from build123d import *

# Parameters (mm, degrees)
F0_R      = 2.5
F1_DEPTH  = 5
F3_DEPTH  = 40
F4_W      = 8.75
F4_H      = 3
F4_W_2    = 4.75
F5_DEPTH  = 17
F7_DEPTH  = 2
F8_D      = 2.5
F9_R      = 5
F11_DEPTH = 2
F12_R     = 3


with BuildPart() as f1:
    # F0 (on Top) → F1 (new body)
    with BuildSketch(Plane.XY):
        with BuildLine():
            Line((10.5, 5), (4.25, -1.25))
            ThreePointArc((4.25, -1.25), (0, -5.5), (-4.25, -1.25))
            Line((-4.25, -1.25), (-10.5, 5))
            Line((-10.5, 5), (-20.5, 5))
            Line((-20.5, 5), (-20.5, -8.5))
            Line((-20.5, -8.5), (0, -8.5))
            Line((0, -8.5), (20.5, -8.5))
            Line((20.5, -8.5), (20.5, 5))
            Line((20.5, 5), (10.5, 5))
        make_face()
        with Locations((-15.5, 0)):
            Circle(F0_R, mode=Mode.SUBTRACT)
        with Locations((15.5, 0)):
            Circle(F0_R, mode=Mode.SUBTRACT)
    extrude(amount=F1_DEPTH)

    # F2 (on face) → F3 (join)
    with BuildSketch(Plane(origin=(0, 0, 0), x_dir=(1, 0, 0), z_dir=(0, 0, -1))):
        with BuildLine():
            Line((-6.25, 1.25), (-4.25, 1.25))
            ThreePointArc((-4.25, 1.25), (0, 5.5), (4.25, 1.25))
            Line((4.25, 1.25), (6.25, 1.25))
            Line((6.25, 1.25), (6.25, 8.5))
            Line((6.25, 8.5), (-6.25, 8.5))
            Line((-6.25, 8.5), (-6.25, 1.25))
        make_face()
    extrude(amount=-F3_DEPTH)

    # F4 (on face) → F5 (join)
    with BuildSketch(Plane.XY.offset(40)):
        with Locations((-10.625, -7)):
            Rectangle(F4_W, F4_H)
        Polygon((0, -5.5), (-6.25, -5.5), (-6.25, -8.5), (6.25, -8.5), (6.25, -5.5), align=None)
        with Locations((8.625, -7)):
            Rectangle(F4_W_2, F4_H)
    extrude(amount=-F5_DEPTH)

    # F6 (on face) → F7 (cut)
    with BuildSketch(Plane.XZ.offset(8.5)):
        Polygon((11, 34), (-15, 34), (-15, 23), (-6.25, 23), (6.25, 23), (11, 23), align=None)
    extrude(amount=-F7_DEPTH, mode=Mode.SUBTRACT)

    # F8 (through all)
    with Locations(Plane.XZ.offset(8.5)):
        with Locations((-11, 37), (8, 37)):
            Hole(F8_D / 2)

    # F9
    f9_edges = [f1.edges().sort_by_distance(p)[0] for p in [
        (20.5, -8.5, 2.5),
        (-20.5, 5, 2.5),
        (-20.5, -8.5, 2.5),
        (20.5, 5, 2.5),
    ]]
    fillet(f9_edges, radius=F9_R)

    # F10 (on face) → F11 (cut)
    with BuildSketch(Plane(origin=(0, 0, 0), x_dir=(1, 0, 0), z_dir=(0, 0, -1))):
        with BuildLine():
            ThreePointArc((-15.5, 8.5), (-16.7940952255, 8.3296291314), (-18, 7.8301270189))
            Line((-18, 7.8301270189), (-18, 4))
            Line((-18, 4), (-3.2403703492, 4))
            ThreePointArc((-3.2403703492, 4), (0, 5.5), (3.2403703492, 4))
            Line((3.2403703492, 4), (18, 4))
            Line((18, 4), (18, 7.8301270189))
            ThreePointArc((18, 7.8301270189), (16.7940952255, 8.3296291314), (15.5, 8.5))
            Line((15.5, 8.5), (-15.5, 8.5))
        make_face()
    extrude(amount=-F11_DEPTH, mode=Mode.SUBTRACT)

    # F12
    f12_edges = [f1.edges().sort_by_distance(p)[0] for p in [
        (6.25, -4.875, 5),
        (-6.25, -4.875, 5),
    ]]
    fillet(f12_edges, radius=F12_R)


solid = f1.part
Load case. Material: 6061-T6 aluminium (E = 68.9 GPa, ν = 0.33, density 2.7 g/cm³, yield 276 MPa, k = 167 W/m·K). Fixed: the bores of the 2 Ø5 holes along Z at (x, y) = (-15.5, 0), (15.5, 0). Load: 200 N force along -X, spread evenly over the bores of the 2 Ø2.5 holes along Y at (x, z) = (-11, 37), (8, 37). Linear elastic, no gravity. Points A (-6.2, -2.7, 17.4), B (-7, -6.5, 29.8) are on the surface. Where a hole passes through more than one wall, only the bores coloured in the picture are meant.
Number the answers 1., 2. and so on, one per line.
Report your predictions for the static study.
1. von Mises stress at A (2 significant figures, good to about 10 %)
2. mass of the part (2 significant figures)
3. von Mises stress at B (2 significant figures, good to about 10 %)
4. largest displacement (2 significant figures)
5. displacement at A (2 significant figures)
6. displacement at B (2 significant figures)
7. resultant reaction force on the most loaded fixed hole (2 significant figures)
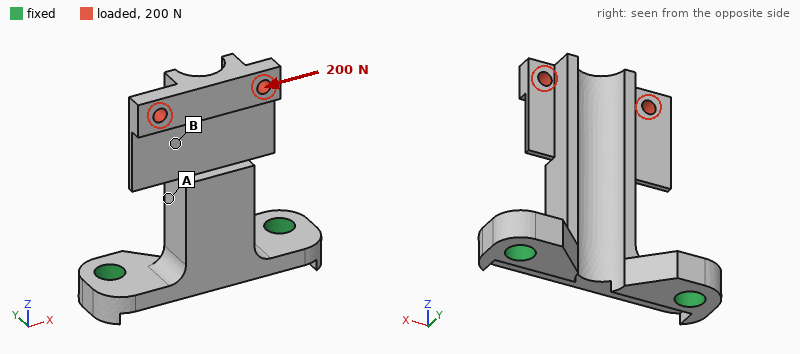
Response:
1. 26 MPa
2. 10 g
3. 9.3 MPa
4. 99 µm
5. 27 µm
6. 60 µm
7. 380 N
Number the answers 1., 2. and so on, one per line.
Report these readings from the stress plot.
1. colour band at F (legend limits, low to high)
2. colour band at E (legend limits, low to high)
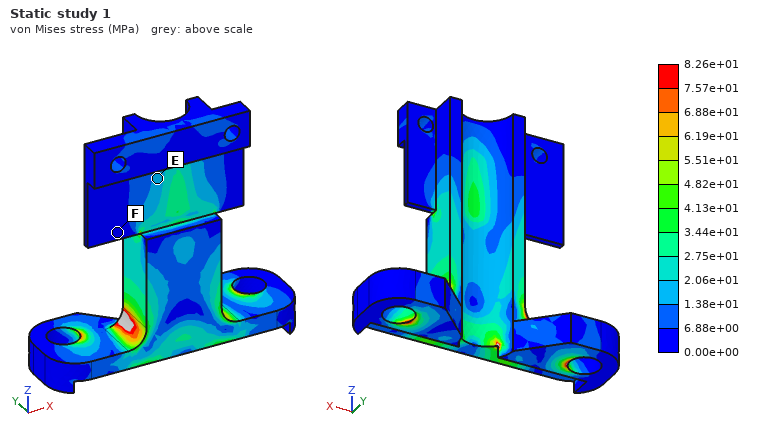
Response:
1. 0.00e+00 to 6.88e+00 MPa
2. 1.38e+01 to 2.06e+01 MPa
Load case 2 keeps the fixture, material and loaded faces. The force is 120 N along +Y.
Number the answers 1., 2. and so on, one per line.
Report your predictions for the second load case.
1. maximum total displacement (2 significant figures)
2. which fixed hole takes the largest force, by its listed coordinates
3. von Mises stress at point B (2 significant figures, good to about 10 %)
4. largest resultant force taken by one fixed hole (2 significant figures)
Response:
1. 0.30 mm
2. (-15.5, 0)
3. 16 MPa
4. 69 N
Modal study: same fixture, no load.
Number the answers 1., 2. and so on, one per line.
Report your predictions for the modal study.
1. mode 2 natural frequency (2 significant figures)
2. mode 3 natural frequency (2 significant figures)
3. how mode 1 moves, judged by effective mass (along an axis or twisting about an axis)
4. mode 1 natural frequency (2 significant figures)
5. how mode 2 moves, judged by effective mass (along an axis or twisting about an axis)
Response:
1. 4600 Hz
2. 5500 Hz
3. along Y
4. 2200 Hz
5. along X
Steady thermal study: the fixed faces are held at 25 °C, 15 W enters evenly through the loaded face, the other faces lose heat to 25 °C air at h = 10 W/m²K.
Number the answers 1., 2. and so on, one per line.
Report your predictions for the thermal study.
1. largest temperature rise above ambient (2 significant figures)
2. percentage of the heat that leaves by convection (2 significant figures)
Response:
1. 71 K
2. 6.4 %
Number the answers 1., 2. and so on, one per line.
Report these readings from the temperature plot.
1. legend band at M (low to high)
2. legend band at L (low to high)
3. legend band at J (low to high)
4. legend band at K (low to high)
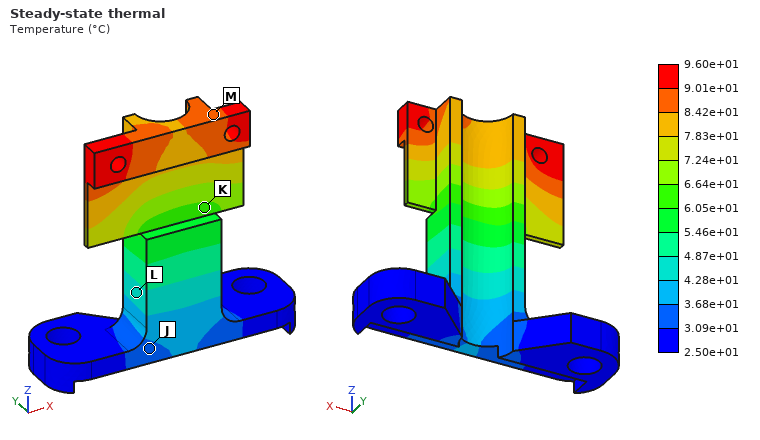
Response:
1. 8.42e+01 to 9.01e+01 °C
2. 4.28e+01 to 4.87e+01 °C
3. 3.09e+01 to 3.68e+01 °C
4. 6.05e+01 to 6.64e+01 °C
